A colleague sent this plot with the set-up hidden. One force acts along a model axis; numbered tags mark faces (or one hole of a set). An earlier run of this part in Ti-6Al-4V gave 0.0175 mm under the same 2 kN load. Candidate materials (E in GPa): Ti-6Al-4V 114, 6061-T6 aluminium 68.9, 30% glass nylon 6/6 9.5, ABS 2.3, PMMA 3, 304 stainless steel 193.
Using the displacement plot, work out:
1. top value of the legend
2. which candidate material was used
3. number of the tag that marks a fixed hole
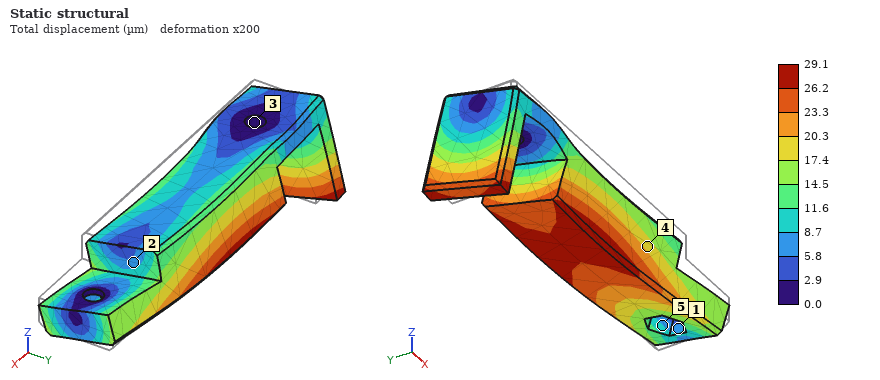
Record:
29.1 µm
6061-T6 aluminium
3
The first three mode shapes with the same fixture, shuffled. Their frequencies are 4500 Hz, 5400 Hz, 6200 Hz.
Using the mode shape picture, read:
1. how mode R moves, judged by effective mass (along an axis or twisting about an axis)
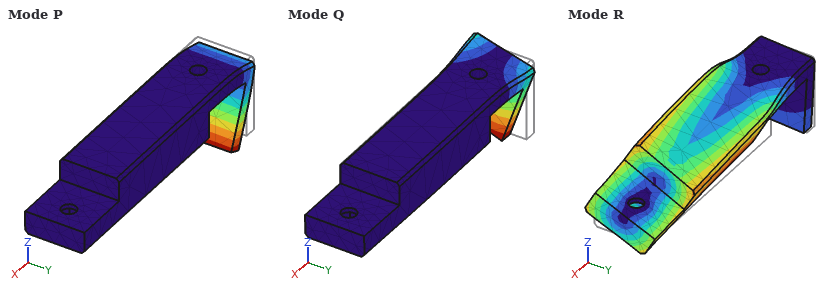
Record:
along Y
